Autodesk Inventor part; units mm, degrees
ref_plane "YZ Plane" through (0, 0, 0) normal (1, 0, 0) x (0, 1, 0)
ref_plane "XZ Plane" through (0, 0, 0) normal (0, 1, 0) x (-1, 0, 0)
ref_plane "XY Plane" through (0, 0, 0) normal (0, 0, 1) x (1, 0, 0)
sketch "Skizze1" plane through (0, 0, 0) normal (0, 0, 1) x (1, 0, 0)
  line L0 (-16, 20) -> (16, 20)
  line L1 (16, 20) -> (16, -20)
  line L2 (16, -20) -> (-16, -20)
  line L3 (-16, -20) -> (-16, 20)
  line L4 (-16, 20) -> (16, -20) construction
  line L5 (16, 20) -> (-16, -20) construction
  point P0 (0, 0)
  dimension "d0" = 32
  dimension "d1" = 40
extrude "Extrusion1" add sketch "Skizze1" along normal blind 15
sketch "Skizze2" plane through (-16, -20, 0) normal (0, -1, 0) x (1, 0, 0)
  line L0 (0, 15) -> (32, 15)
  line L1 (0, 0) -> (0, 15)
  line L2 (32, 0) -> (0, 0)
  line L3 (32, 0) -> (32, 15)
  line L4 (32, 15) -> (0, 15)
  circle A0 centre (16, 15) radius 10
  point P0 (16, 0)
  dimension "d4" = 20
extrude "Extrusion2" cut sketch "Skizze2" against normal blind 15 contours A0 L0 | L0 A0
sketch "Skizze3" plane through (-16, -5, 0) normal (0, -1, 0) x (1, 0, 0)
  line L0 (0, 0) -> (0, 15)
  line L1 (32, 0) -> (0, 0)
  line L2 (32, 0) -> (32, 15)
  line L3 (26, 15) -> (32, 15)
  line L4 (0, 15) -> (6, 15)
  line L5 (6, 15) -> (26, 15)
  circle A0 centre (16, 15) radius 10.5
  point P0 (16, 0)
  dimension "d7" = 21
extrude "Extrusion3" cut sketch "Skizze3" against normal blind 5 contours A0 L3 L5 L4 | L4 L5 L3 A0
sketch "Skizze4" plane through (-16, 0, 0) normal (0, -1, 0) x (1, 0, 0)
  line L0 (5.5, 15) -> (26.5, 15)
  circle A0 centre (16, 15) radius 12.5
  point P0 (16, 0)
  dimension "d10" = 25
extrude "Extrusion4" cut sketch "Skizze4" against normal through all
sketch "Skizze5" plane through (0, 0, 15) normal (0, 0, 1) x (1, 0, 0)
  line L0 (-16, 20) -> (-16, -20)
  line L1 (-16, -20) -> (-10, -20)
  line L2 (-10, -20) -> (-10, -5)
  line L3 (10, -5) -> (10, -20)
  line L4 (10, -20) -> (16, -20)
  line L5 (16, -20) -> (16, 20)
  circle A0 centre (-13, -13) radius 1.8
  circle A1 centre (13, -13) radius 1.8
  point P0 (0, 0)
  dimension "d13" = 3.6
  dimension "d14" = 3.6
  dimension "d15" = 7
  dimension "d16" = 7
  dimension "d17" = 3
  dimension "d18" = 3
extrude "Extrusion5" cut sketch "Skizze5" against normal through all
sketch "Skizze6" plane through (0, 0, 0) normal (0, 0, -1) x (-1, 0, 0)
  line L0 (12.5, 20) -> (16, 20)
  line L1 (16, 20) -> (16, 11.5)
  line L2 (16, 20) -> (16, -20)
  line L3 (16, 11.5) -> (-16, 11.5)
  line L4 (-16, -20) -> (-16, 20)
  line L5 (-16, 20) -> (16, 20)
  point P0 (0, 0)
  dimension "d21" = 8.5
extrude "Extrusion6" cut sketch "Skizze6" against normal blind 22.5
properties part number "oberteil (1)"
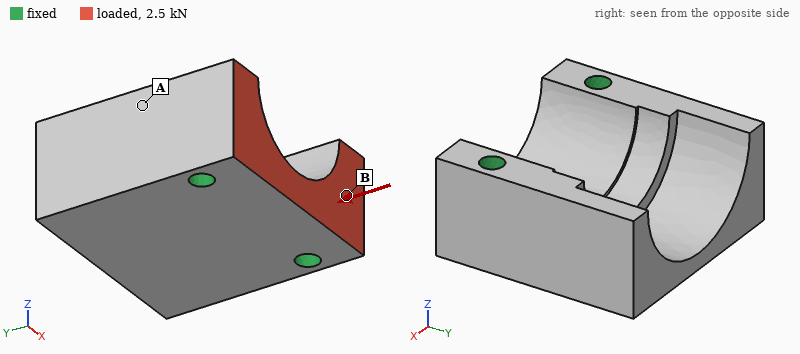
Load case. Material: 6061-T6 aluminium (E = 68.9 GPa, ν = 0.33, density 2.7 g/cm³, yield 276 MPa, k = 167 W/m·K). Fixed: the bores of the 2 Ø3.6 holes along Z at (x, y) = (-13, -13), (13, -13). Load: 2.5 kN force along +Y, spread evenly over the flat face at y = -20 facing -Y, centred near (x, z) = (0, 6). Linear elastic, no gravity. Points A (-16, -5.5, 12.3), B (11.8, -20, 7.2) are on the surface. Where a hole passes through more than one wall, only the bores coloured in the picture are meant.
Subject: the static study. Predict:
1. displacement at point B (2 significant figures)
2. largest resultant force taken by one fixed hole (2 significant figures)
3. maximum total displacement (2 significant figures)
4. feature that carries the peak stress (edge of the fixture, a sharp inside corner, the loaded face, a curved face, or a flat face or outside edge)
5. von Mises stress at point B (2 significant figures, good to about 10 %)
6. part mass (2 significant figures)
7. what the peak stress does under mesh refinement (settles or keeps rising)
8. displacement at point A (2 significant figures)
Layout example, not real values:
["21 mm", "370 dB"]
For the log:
["1.0 µm", "1.3 kN", "2.8 µm", "edge of the fixture", "9.1 MPa", "24 g", "keeps rising", "0.46 µm"]
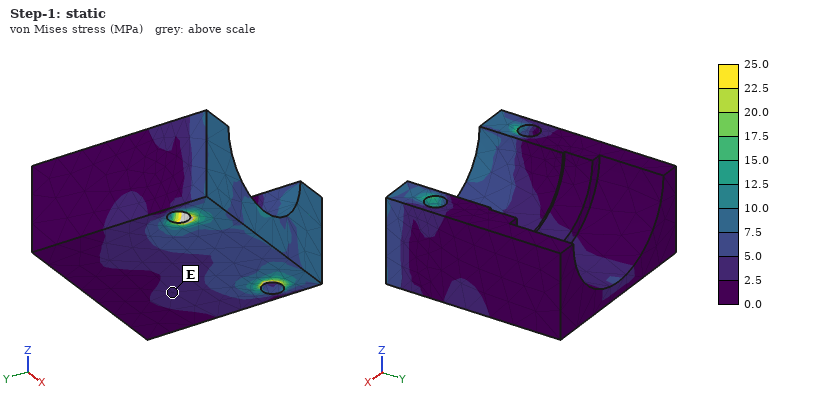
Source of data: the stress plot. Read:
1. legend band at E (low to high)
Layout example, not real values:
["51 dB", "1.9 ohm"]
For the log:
["2.5 to 5.0 MPa"]
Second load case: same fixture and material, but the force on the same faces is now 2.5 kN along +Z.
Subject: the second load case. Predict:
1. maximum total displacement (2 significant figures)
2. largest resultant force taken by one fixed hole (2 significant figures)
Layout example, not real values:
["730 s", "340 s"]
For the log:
["8.8 µm", "1.3 kN"]
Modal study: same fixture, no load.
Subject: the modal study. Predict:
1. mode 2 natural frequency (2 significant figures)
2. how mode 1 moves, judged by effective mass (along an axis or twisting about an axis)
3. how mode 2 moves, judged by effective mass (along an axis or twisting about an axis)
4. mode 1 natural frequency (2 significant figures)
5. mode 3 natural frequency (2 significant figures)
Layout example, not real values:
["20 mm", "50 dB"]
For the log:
["17 kHz", "along Z", "along X", "16 kHz", "21 kHz"]
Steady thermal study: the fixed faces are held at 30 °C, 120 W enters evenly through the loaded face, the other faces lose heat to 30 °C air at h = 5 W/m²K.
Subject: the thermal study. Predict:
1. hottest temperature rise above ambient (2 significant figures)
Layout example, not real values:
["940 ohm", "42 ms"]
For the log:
["22 K"]
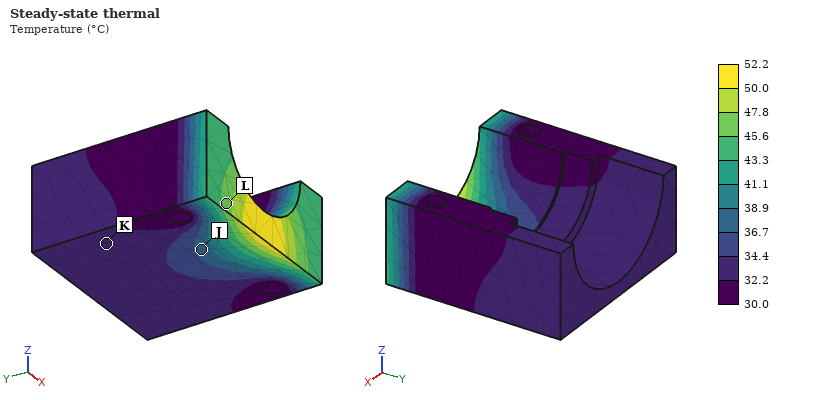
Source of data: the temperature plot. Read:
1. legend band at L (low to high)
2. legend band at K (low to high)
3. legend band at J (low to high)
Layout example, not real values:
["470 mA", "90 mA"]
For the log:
["45.6 to 47.8 °C", "32.2 to 34.4 °C", "36.7 to 38.9 °C"]
